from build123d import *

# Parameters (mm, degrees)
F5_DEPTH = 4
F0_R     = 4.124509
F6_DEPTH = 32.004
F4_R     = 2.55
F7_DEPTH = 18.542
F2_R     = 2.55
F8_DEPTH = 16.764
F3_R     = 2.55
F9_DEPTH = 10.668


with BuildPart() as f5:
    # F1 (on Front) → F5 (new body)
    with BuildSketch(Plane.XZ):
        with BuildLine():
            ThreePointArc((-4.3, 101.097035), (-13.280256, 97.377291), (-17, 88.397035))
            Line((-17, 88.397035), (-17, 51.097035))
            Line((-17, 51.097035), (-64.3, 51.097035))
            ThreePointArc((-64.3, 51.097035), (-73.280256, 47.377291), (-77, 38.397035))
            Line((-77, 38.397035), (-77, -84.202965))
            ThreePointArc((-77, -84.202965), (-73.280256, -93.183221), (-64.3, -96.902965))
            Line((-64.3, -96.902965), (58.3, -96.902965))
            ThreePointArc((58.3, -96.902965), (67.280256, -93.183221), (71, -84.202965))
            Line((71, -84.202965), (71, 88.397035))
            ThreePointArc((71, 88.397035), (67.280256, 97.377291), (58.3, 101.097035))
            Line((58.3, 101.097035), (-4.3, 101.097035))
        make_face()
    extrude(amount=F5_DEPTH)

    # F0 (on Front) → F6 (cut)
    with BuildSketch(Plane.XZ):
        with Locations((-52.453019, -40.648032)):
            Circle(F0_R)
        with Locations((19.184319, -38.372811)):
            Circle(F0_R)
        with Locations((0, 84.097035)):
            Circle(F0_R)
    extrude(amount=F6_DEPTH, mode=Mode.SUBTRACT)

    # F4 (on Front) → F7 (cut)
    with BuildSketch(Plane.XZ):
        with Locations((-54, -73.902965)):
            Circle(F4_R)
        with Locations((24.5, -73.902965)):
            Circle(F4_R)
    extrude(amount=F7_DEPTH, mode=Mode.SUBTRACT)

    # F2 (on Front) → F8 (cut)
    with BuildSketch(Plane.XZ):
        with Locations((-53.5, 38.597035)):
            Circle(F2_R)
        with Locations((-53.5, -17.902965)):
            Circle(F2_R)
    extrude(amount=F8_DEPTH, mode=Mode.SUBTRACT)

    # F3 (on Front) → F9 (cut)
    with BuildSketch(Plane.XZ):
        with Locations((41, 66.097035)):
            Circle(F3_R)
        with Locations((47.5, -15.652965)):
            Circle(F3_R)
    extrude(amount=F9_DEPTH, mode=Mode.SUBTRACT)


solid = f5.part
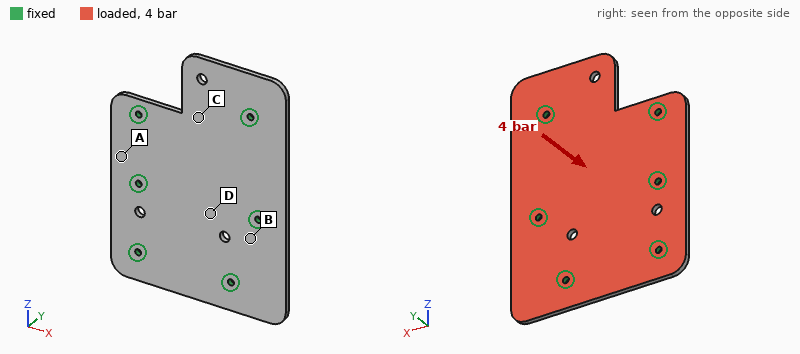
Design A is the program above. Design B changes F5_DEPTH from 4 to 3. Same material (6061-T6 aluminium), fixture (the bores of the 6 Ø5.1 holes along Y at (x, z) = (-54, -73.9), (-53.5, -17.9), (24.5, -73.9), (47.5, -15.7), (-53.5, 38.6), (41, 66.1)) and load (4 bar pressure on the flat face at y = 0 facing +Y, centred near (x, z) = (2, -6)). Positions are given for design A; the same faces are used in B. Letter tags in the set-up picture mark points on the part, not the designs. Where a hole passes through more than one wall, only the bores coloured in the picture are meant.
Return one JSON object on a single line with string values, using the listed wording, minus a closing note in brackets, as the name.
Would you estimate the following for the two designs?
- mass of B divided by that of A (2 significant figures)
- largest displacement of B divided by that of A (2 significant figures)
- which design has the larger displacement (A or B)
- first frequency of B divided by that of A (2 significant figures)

{"mass of B divided by that of A": "0.75", "largest displacement of B divided by that of A": "2.3", "which design has the larger displacement": "B", "first frequency of B divided by that of A": "0.76"}
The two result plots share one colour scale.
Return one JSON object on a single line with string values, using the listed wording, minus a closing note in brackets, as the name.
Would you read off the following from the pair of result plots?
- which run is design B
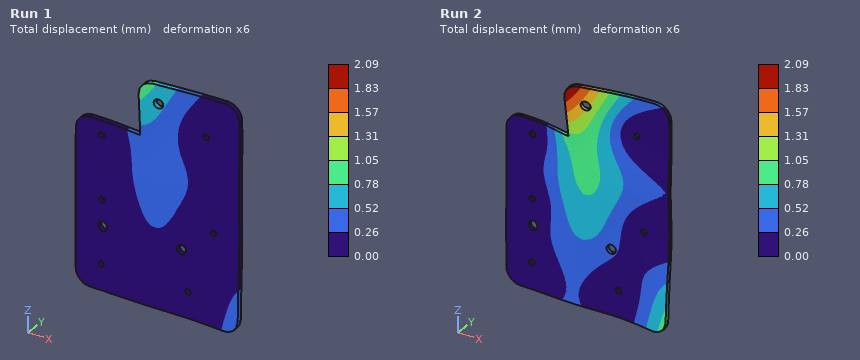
{"which run is design B": "Run 2"}
